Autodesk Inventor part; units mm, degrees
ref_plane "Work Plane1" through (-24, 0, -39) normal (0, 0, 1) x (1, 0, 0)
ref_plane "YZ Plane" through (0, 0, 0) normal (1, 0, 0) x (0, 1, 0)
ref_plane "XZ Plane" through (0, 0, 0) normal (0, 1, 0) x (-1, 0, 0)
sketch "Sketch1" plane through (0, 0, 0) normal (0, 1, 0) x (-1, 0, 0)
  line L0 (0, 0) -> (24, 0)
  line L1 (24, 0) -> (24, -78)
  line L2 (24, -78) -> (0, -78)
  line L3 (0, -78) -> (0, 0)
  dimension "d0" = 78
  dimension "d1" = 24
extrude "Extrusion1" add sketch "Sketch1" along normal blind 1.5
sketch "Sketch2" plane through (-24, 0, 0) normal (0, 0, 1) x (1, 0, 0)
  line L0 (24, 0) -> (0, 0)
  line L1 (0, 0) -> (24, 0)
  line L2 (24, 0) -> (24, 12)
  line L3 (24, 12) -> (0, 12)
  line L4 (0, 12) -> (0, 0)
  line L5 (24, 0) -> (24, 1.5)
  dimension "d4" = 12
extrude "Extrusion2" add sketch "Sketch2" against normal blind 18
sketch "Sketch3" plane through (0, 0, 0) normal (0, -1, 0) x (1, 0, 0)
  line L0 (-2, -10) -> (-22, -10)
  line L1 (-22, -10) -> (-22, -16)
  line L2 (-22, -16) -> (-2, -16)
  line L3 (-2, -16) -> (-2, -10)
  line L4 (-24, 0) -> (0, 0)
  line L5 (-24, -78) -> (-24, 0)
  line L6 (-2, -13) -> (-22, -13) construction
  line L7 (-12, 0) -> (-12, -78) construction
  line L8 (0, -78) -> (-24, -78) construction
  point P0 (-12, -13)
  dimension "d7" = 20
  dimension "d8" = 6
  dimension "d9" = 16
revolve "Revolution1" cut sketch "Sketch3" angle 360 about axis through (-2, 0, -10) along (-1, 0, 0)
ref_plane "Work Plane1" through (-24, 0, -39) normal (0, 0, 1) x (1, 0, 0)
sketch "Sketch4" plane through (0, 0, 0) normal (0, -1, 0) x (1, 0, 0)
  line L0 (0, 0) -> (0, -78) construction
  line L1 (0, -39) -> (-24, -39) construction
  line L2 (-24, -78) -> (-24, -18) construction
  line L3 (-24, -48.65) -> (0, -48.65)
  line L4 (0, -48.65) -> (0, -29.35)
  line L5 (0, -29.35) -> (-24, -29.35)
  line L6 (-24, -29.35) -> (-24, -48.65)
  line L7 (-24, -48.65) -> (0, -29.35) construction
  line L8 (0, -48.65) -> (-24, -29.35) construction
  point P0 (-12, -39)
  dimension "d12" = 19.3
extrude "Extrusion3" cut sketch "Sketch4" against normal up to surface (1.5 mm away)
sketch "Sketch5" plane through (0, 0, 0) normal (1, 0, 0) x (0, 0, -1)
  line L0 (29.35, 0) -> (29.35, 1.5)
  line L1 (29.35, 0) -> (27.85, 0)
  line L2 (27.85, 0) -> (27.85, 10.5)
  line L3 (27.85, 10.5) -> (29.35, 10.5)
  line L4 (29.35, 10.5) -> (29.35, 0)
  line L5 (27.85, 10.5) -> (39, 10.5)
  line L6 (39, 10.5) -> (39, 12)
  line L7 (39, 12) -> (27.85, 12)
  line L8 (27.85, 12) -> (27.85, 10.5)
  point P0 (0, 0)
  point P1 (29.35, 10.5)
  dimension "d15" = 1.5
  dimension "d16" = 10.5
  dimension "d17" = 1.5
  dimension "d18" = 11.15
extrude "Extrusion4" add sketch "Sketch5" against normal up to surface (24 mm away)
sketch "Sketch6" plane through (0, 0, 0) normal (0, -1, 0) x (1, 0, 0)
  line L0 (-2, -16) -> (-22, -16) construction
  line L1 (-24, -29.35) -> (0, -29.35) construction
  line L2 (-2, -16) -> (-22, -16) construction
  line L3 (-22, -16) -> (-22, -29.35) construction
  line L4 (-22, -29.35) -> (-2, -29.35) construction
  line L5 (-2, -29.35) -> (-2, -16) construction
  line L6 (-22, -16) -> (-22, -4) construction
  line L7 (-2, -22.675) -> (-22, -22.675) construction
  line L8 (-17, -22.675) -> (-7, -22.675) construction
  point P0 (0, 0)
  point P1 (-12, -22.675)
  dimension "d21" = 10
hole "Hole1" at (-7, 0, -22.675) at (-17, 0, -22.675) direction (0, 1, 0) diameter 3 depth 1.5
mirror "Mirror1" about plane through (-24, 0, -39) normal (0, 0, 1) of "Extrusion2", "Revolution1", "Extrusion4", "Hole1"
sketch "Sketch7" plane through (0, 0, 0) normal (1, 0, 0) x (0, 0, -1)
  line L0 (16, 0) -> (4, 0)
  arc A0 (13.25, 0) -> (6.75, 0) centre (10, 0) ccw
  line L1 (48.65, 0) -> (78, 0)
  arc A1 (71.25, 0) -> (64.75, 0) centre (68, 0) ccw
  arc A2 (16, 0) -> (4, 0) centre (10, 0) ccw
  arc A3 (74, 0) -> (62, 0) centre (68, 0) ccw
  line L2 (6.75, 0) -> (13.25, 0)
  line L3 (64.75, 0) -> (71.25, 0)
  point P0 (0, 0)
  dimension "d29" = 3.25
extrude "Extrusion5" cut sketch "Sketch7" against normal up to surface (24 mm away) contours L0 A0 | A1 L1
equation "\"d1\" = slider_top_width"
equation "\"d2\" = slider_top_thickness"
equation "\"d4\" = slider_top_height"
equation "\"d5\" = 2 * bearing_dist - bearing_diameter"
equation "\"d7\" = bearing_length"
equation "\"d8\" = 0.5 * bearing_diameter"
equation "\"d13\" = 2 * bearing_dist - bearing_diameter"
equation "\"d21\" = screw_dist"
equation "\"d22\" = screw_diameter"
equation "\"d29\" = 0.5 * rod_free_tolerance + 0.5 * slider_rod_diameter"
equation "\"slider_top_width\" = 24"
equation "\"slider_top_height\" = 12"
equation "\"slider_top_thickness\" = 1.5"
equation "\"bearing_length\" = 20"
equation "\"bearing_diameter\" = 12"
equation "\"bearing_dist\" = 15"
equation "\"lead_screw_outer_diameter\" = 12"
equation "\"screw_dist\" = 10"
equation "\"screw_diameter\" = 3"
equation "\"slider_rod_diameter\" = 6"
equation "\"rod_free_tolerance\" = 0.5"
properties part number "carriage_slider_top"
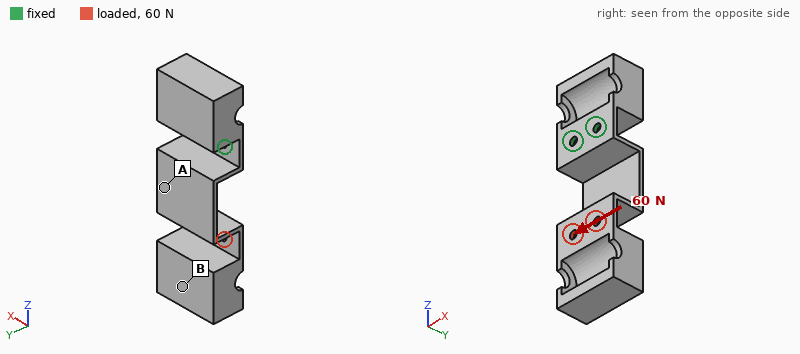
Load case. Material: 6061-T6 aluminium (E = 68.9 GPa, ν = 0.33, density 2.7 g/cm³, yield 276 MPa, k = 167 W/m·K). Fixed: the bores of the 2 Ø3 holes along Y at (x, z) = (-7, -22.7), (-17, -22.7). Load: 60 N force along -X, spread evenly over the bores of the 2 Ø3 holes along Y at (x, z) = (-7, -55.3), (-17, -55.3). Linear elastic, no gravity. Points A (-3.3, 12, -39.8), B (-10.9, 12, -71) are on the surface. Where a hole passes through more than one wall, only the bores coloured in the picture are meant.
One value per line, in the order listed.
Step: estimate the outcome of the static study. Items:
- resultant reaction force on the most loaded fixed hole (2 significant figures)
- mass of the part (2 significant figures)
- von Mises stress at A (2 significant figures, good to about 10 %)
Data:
160 N
28 g
57 MPa
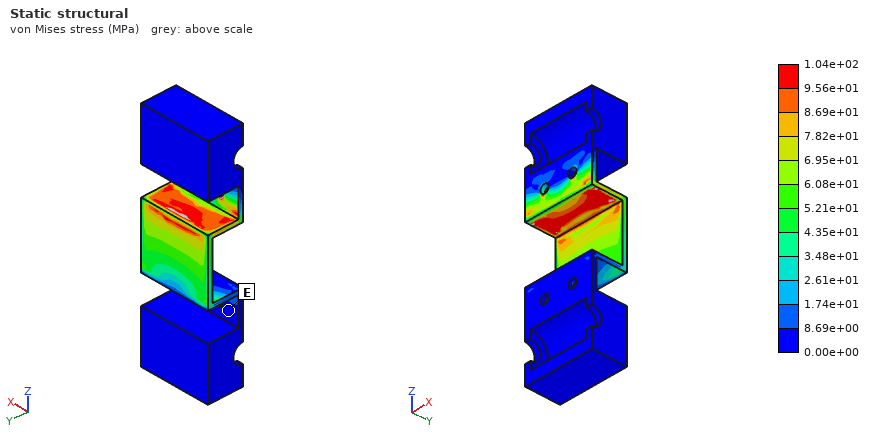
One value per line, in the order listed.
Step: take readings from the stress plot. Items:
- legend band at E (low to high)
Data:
0.00e+00 to 8.69e+00 MPa
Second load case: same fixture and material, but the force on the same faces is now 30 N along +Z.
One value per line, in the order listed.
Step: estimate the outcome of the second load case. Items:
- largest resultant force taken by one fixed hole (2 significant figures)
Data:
15 N
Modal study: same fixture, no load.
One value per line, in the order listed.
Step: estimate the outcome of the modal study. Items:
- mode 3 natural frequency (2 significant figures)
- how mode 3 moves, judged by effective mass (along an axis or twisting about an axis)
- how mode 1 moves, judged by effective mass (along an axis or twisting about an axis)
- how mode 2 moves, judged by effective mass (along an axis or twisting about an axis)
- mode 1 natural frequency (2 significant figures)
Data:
900 Hz
along Z
along Y
along X
140 Hz
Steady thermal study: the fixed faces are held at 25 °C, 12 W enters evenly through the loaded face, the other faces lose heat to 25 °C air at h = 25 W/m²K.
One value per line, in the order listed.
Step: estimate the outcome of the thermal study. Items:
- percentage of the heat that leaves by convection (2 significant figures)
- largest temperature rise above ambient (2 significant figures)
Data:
45 %
65 K
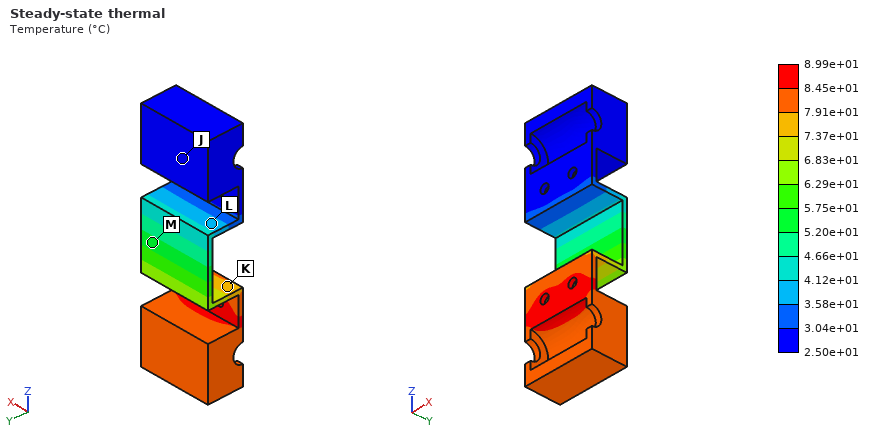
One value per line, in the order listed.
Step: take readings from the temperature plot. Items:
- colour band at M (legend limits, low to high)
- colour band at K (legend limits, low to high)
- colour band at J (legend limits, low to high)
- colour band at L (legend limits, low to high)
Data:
5.20e+01 to 5.75e+01 °C
7.37e+01 to 7.91e+01 °C
2.50e+01 to 3.04e+01 °C
3.58e+01 to 4.12e+01 °C
